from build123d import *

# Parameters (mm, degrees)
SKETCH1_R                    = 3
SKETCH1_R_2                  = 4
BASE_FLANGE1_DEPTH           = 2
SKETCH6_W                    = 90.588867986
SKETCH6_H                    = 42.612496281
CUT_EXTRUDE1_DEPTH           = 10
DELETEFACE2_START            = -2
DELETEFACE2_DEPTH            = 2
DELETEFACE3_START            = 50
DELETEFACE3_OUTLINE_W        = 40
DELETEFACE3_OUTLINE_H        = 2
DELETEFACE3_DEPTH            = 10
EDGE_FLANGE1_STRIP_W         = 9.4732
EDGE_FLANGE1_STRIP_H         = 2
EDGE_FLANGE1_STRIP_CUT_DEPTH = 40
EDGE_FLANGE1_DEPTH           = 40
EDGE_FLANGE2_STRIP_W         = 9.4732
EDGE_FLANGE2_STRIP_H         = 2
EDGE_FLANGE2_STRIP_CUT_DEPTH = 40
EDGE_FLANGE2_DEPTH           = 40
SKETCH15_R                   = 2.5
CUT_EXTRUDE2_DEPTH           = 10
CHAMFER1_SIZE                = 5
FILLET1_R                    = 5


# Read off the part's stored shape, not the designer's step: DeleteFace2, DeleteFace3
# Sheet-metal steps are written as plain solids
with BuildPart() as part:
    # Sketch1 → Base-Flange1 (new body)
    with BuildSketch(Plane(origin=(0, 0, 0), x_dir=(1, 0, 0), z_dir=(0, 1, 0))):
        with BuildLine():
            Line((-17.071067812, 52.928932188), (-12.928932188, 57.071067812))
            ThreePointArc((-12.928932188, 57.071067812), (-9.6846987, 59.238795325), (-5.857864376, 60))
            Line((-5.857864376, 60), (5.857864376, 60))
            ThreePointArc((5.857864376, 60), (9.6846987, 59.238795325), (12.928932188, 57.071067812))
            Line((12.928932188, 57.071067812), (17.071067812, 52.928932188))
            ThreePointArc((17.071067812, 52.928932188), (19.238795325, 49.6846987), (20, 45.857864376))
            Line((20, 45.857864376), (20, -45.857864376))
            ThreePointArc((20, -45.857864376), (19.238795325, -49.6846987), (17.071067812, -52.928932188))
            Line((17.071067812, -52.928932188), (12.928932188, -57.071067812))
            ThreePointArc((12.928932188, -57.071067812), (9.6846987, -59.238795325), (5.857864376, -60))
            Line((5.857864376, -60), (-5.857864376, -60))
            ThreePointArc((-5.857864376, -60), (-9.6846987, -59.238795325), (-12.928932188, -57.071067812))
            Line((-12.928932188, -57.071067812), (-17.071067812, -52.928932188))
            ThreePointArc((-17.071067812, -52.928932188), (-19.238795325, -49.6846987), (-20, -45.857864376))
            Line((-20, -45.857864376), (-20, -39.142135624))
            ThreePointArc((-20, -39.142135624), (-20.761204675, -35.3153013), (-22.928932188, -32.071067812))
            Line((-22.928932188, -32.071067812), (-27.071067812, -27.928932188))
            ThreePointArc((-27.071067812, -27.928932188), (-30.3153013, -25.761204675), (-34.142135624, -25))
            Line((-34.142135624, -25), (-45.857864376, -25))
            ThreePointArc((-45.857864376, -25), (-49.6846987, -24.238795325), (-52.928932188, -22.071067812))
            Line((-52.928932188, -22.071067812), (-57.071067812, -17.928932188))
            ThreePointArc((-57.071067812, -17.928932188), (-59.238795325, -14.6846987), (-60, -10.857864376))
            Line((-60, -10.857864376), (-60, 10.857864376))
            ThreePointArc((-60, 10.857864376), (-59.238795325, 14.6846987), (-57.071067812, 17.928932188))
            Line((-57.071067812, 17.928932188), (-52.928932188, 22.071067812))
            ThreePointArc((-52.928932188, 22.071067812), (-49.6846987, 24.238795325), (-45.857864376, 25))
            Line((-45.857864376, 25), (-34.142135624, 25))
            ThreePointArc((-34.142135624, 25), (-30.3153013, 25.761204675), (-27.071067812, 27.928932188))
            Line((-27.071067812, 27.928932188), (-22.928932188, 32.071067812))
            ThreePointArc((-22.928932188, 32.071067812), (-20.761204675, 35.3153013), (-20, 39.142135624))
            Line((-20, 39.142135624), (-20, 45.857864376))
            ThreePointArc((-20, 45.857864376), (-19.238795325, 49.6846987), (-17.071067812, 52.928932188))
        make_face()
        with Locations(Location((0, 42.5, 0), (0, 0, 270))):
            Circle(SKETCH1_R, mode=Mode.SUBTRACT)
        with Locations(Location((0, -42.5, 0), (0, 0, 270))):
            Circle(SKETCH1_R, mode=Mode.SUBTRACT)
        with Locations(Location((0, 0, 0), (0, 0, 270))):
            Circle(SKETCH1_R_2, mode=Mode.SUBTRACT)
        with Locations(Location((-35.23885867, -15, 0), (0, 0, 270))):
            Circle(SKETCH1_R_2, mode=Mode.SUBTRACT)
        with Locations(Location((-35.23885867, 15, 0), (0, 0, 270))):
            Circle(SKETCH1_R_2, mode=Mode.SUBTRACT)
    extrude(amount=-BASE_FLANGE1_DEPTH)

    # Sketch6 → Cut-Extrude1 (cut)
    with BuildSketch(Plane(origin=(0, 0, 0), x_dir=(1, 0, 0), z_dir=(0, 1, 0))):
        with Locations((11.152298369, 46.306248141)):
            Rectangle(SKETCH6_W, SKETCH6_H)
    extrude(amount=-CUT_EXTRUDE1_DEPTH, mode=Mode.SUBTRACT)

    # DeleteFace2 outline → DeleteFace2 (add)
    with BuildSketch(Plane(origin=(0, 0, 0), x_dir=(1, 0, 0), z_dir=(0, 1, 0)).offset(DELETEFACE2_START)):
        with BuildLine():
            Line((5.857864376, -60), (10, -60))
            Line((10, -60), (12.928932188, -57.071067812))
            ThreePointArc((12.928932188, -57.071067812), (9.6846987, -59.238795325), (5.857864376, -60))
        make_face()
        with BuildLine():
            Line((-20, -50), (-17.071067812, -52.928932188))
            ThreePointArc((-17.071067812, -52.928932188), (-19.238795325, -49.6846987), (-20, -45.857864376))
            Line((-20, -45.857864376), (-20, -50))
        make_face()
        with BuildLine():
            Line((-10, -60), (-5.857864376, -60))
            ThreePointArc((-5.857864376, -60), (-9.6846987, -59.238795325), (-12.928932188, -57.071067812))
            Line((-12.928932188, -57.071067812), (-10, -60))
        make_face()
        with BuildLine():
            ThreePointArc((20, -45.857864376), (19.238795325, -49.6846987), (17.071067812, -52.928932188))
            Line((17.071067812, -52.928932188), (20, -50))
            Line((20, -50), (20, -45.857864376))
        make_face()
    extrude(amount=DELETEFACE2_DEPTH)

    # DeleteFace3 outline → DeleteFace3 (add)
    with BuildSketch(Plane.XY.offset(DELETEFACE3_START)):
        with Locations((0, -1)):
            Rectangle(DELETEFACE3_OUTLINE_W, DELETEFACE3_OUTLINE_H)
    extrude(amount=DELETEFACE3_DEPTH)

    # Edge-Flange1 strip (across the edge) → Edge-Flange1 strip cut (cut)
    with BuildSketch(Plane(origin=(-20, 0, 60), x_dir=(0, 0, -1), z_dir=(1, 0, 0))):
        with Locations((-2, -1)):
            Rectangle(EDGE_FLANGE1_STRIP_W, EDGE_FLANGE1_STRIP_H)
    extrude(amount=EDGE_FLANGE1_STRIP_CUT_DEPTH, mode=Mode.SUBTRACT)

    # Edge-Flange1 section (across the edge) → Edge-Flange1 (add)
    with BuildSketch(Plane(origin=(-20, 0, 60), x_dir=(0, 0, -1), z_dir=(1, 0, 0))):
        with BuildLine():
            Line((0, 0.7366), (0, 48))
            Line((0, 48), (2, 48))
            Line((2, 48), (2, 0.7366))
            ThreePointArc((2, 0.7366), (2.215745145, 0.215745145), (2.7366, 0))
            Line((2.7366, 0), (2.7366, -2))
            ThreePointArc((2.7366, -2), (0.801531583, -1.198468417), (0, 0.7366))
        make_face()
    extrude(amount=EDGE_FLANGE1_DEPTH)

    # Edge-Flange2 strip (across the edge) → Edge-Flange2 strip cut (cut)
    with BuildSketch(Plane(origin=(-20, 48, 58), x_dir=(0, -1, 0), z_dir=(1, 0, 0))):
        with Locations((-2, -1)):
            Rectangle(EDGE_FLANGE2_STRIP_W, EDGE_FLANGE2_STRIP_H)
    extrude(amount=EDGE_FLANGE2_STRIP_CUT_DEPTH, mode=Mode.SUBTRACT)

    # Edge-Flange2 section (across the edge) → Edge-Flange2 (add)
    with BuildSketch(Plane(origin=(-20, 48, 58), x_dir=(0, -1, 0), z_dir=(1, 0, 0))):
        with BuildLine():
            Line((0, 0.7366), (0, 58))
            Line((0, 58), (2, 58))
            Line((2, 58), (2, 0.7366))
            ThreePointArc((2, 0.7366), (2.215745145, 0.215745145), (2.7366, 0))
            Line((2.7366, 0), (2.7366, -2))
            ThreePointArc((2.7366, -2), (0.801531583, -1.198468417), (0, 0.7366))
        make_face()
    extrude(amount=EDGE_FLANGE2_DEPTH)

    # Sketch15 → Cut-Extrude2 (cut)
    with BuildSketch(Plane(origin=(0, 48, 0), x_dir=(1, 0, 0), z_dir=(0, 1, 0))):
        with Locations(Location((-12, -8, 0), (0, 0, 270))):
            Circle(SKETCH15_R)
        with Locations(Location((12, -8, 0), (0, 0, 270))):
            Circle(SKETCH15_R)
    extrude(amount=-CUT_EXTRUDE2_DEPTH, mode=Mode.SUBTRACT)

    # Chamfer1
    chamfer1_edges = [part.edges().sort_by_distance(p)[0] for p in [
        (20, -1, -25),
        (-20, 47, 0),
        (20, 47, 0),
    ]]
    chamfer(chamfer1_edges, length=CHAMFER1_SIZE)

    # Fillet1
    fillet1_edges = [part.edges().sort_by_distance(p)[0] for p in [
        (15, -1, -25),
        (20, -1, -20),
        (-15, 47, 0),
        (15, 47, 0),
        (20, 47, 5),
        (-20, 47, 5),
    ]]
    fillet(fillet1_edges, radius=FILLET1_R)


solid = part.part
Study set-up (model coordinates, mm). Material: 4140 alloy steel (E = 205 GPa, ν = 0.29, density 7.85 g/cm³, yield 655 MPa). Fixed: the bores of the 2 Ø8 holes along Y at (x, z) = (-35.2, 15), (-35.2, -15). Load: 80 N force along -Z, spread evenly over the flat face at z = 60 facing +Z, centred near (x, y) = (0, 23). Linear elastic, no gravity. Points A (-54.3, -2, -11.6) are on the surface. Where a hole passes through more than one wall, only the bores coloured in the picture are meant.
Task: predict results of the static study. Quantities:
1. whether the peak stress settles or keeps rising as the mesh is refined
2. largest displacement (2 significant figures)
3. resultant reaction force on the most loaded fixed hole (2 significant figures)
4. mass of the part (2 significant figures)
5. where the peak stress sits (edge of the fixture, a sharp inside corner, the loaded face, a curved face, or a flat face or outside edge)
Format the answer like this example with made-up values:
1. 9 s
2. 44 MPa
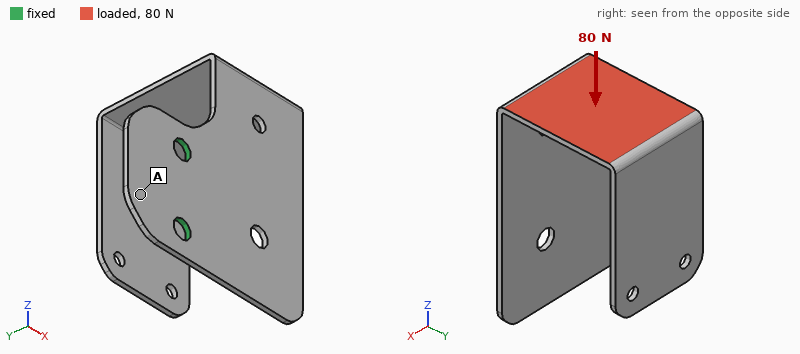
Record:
1. keeps rising
2. 1.4 mm
3. 95 N
4. 150 g
5. a sharp inside corner
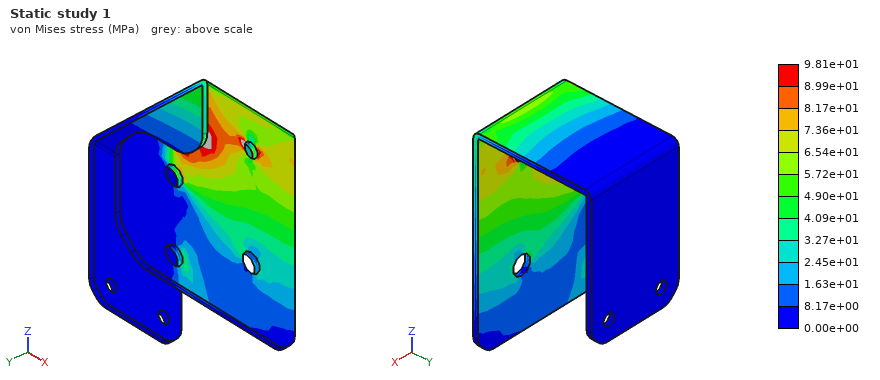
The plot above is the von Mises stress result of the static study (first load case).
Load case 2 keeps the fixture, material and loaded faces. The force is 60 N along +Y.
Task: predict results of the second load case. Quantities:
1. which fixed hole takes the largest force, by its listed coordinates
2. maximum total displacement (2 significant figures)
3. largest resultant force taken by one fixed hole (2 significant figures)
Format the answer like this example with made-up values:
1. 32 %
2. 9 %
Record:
1. (-35.2, 15)
2. 1.2 mm
3. 110 N
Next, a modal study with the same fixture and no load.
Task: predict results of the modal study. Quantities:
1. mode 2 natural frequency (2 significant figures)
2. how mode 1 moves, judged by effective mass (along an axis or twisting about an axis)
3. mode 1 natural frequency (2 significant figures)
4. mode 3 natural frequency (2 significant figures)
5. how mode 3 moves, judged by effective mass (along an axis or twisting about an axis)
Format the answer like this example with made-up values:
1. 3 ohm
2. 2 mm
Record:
1. 150 Hz
2. along Z
3. 120 Hz
4. 250 Hz
5. along Y
